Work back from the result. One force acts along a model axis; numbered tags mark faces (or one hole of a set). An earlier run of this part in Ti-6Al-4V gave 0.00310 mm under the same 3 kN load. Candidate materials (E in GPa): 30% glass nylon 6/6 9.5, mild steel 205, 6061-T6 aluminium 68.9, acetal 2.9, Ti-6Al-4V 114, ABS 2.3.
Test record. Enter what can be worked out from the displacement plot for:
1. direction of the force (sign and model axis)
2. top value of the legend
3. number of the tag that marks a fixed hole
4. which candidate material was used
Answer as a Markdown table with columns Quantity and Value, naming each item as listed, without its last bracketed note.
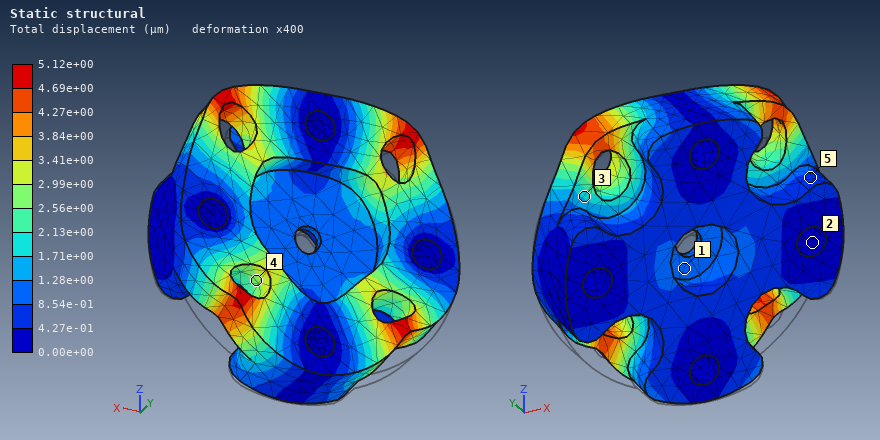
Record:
| Quantity | Value |
|---|---|
| direction of the force | +Z |
| top value of the legend | 5.12e+00 µm |
| number of the tag that marks a fixed hole | 2 |
| which candidate material was used | 6061-T6 aluminium |
